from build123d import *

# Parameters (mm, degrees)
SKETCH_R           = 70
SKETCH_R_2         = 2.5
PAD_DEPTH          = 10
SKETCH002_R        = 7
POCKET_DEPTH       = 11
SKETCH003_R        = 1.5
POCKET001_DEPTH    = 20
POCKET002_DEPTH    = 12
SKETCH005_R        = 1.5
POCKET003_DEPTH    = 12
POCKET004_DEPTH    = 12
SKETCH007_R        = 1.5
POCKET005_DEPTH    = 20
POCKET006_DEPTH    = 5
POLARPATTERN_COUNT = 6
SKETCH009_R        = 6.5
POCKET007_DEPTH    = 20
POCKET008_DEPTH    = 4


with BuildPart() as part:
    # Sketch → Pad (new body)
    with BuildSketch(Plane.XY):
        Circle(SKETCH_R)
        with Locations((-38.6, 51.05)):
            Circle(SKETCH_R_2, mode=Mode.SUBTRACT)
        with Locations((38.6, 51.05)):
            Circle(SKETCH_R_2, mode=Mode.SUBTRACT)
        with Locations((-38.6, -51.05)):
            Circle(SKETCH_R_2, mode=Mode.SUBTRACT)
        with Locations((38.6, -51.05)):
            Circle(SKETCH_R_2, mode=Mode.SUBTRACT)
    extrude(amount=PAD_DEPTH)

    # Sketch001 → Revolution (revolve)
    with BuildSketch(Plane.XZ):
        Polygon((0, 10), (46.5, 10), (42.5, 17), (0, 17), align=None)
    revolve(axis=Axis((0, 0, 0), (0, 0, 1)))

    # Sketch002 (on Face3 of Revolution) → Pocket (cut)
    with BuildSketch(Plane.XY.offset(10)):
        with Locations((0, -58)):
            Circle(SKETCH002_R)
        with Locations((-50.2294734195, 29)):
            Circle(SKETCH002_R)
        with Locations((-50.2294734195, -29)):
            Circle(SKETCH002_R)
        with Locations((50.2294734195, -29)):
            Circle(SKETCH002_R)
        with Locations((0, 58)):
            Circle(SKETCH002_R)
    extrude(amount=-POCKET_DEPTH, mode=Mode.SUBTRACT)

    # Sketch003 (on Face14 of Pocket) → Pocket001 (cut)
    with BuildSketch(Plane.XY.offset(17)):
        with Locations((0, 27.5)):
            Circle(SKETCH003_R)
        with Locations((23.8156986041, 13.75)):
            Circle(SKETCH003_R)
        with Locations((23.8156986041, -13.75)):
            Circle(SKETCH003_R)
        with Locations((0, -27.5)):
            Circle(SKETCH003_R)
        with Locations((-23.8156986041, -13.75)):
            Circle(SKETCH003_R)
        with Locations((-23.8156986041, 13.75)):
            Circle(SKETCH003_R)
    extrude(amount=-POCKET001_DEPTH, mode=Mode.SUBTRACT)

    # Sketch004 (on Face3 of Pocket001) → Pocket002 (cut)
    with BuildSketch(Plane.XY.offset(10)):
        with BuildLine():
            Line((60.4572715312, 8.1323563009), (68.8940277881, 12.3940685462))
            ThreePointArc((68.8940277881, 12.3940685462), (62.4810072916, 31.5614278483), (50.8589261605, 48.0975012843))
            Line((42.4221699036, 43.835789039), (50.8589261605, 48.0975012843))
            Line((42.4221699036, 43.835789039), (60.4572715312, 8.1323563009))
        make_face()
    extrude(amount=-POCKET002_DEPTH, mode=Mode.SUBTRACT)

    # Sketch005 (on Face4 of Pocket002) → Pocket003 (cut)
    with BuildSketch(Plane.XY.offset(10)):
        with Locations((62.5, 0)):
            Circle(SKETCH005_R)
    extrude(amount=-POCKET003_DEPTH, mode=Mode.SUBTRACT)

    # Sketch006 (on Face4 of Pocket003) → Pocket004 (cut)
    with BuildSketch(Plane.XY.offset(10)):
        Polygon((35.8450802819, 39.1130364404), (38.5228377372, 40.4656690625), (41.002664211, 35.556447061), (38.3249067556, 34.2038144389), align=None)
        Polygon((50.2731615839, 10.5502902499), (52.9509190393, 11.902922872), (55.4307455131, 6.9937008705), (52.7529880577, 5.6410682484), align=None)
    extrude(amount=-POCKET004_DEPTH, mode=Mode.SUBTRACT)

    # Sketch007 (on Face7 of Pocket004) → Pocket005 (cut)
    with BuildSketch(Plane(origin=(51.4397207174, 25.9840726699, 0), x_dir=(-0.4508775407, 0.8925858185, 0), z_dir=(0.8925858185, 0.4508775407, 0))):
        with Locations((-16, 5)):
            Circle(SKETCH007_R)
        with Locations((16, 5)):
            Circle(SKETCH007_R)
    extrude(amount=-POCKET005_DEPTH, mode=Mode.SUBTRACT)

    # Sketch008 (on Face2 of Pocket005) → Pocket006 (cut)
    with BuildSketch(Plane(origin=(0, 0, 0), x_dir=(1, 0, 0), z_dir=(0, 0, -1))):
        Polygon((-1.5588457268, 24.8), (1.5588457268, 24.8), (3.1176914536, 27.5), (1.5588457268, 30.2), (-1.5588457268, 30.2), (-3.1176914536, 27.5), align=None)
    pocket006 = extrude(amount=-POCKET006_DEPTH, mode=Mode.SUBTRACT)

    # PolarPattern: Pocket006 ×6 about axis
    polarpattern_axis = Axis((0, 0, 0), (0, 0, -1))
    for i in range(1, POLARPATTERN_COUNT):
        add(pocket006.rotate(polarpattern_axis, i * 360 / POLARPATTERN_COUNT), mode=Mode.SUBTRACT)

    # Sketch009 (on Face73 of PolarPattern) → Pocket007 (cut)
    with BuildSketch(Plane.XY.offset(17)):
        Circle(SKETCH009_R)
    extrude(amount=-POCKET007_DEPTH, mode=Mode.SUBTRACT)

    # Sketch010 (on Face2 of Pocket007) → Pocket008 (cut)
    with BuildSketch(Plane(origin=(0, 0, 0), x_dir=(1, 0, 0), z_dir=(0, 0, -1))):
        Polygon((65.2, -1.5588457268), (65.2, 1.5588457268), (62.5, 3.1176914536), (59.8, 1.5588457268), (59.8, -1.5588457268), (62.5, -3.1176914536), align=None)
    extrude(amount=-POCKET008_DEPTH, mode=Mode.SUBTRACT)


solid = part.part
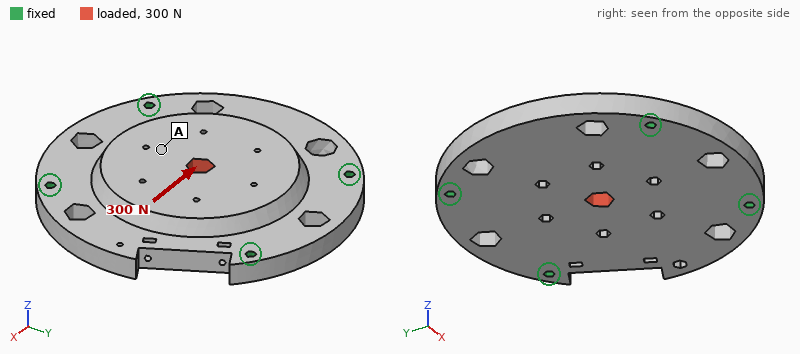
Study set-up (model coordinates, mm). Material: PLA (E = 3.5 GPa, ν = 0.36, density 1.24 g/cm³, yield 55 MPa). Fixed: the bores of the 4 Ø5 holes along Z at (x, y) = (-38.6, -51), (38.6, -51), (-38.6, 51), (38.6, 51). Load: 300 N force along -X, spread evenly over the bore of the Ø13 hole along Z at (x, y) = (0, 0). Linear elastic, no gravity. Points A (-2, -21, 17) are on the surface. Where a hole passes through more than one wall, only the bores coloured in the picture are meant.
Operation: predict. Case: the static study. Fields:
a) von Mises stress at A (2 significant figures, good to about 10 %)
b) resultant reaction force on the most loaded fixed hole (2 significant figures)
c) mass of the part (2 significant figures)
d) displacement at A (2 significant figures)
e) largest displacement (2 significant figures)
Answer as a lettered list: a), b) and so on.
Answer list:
a) 0.18 MPa
b) 84 N
c) 220 g
d) 4.8 µm
e) 7.5 µm
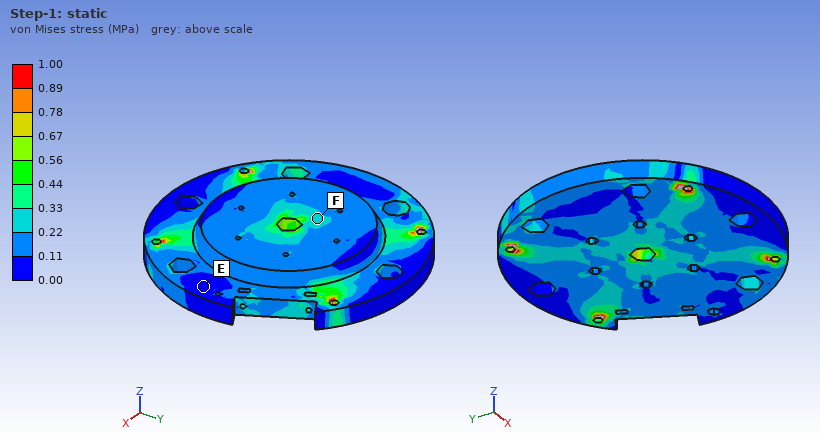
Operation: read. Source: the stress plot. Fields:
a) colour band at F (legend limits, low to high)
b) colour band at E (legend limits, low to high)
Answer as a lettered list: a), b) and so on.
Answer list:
a) 0.22 to 0.33 MPa
b) 0.00 to 0.11 MPa
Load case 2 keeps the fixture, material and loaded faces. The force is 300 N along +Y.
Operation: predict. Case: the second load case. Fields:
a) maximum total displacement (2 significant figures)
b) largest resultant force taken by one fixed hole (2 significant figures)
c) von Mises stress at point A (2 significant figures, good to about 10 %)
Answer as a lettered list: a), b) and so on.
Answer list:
a) 5.9 µm
b) 81 N
c) 0.18 MPa
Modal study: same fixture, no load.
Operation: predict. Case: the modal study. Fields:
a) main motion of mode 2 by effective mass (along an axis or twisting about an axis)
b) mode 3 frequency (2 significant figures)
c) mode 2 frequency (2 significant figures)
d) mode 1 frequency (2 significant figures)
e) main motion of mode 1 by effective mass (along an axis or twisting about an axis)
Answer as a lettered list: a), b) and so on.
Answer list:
a) twisting about Y
b) 2000 Hz
c) 1400 Hz
d) 1300 Hz
e) along Z
